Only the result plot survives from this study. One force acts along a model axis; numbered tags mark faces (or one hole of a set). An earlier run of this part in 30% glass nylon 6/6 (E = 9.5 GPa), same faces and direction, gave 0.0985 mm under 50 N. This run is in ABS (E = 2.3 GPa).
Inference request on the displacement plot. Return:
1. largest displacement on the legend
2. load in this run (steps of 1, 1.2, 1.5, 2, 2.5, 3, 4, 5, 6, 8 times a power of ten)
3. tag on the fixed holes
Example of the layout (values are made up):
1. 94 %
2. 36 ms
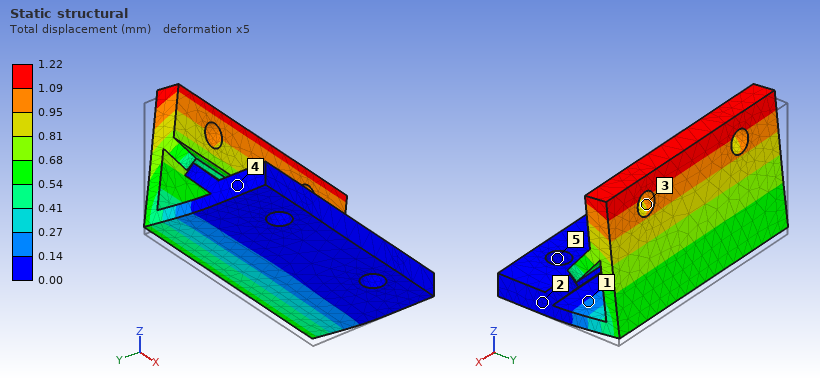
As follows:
1. 1.22 mm
2. 150 N
3. 5
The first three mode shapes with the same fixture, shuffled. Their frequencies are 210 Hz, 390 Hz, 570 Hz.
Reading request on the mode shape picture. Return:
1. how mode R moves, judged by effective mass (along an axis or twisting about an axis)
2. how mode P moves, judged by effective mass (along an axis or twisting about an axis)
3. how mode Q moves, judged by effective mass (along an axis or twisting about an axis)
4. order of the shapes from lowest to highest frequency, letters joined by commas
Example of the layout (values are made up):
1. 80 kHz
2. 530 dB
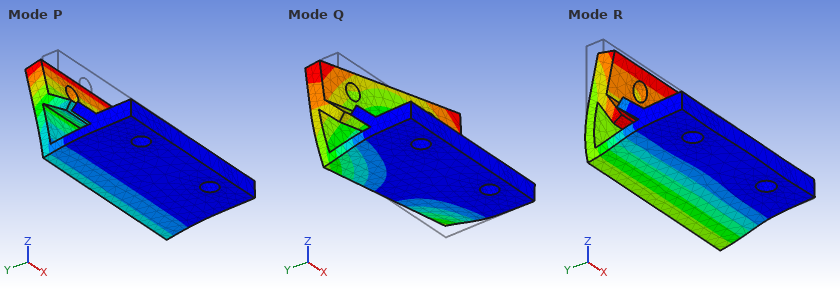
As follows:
1. along Z
2. along Y
3. along X
4. P, Q, R
